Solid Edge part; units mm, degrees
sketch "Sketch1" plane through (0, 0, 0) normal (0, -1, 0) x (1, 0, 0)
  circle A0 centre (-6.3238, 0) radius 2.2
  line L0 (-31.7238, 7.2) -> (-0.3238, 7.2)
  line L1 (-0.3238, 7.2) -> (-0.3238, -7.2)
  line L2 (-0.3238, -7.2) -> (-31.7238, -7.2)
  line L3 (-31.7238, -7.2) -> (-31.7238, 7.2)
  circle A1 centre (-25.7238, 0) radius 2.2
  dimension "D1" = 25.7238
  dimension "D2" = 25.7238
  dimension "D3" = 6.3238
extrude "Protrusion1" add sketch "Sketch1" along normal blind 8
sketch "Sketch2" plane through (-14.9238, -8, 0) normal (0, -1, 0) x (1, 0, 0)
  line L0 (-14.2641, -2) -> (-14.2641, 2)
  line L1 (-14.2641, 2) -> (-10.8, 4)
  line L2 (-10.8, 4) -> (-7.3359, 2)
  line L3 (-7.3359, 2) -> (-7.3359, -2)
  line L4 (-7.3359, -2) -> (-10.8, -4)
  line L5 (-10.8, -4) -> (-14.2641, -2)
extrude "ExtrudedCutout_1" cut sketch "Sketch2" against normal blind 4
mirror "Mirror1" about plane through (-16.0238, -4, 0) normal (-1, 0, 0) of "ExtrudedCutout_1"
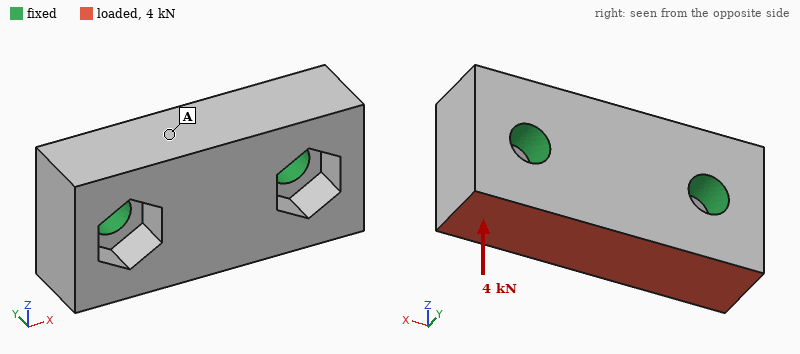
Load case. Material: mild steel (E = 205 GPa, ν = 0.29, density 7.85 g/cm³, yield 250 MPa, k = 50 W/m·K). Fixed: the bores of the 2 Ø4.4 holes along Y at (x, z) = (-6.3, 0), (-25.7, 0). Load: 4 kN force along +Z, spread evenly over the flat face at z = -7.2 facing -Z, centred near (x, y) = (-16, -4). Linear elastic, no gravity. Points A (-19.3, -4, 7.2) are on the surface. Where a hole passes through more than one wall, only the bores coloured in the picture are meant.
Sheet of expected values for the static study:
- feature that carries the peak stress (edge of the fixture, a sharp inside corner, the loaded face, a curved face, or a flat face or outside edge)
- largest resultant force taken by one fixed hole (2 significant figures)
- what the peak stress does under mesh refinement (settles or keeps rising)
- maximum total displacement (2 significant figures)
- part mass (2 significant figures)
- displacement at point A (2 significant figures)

edge of the fixture
2.0 kN
keeps rising
4.5 µm
25 g
2.6 µm
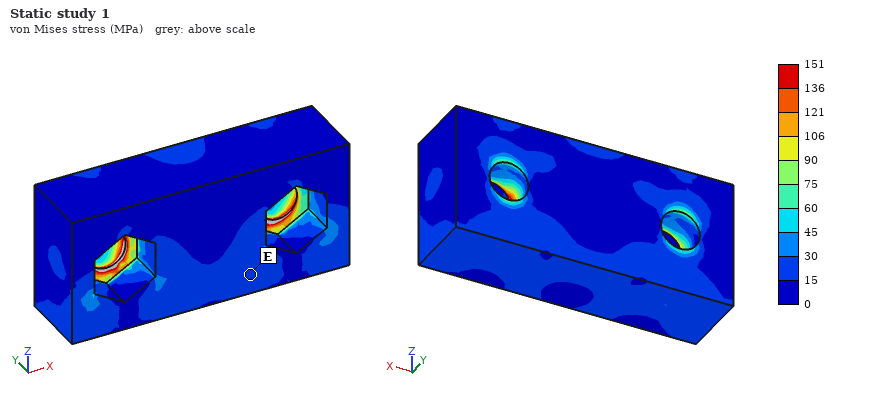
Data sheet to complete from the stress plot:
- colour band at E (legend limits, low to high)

15 to 30 MPa
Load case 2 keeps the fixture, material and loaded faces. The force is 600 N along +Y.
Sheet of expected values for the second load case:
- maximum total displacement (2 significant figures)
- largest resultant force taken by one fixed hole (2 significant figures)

2.1 µm
300 N
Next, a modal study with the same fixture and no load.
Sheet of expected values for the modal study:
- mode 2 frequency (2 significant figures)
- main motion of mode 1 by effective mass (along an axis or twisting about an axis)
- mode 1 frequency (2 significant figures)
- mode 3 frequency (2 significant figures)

47 kHz
along Z
32 kHz
49 kHz
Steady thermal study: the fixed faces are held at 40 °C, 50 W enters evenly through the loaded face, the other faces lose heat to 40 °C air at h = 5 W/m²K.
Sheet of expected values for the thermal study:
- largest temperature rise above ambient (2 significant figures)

46 K
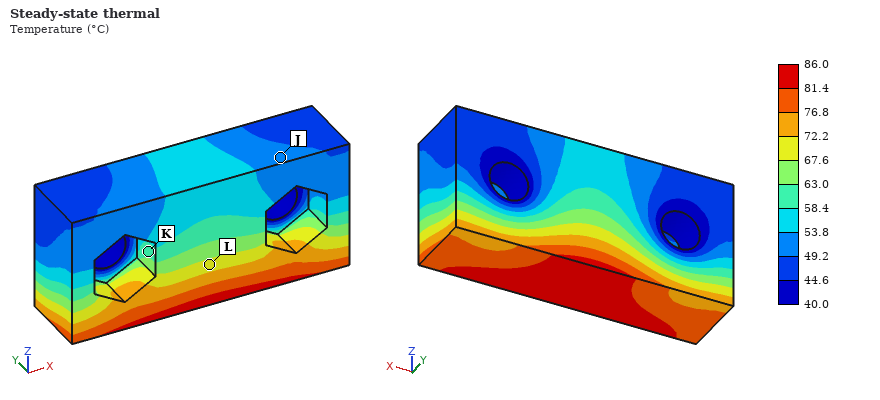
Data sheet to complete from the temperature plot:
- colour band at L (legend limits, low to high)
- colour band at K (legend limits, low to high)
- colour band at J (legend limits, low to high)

67.6 to 72.2 °C
58.4 to 63.0 °C
49.2 to 53.8 °C
